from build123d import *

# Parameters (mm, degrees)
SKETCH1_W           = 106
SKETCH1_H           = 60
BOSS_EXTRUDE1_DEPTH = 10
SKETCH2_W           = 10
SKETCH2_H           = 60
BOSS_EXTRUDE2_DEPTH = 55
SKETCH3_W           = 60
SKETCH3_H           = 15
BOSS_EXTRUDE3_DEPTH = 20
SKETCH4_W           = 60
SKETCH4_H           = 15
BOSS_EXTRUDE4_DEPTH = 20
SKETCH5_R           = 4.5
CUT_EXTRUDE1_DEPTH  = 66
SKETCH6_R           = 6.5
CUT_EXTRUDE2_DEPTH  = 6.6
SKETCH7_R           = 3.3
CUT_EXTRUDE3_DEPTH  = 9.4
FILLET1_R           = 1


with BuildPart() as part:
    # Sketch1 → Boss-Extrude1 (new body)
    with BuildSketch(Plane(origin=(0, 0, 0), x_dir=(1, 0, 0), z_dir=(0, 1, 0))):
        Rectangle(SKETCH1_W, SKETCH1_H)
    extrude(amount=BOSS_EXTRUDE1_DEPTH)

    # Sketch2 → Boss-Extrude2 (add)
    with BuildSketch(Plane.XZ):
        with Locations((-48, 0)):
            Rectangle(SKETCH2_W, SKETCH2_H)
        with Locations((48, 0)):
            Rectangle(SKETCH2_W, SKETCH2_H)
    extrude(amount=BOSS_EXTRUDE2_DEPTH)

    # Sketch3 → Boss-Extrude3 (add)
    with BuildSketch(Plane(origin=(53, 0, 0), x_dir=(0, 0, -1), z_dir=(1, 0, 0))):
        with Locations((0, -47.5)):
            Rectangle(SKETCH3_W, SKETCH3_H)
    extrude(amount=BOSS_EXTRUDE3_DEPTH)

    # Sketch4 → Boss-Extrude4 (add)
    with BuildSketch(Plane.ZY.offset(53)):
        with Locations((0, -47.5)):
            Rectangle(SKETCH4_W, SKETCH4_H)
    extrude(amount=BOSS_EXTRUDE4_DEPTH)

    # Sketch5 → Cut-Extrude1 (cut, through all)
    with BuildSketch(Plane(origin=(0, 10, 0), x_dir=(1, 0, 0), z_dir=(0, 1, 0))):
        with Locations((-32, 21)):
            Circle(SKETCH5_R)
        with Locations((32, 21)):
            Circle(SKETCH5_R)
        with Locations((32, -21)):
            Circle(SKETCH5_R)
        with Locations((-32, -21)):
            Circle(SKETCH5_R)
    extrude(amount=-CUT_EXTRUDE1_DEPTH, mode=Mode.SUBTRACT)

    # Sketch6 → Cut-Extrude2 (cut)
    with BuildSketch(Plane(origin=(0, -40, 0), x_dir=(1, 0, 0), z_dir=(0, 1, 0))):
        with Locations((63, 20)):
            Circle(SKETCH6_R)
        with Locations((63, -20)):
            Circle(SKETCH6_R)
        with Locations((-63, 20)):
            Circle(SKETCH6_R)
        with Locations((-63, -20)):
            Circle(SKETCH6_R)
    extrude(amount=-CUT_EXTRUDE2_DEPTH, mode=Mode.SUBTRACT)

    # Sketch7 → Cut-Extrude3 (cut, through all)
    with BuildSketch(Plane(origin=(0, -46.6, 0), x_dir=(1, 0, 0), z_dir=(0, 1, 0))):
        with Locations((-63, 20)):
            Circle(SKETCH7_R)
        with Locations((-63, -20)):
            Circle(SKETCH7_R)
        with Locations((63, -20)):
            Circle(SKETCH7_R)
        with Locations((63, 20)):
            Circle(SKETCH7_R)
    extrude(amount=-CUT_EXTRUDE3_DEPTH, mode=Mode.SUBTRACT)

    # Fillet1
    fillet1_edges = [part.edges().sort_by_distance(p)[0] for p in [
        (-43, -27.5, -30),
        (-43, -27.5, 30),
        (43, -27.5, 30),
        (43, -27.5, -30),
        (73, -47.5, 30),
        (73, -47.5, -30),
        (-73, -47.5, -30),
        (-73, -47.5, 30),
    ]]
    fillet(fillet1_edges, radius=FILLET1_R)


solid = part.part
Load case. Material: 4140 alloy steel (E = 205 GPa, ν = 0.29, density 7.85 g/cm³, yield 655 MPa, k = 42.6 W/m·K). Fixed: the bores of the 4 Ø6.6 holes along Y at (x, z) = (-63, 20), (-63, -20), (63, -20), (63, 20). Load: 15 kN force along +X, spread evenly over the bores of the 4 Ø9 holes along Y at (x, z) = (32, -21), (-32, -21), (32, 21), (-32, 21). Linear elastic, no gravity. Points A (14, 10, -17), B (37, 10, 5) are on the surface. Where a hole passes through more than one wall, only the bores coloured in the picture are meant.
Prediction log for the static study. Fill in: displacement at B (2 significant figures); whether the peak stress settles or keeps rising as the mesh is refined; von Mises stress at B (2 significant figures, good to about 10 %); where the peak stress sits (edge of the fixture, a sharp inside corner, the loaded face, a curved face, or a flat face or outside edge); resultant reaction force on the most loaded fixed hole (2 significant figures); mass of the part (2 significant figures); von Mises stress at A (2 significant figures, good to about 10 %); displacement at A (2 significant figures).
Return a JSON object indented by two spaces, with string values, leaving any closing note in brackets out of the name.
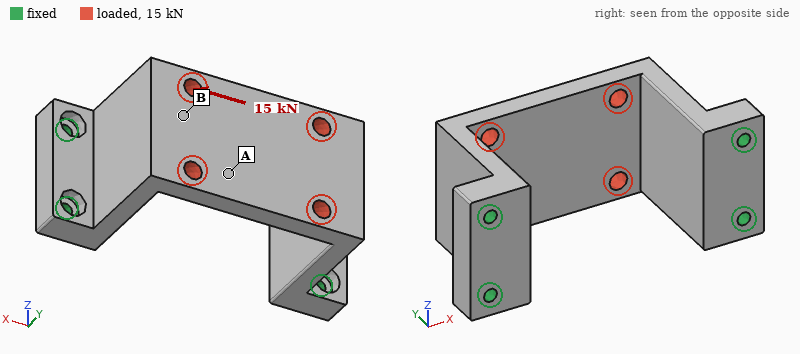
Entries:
{
  "displacement at B": "0.19 mm",
  "whether the peak stress settles or keeps rising as the mesh is refined": "keeps rising",
  "von Mises stress at B": "140 MPa",
  "where the peak stress sits": "edge of the fixture",
  "resultant reaction force on the most loaded fixed hole": "4.4 kN",
  "mass of the part": "1.2 kg",
  "von Mises stress at A": "52 MPa",
  "displacement at A": "0.18 mm"
}
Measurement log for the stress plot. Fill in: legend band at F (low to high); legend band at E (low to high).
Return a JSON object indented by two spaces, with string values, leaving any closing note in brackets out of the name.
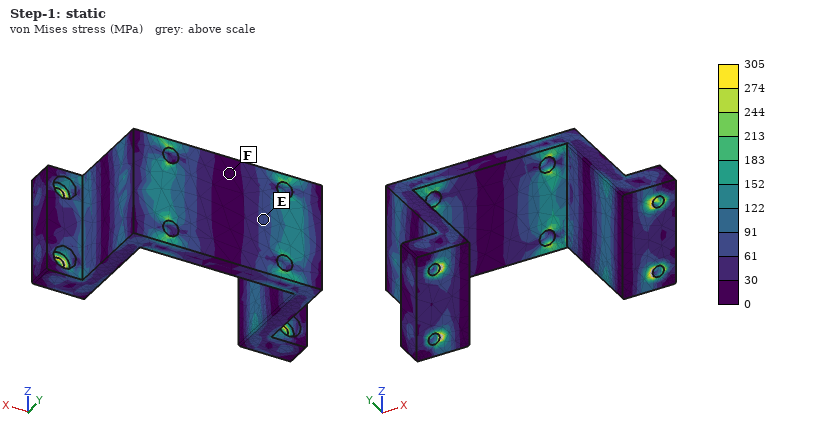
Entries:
{
  "legend band at F": "0 to 30 MPa",
  "legend band at E": "61 to 91 MPa"
}
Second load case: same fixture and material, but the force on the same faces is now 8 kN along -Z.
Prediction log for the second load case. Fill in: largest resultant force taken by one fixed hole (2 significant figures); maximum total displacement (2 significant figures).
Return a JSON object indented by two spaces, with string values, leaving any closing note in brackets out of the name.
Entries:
{
  "largest resultant force taken by one fixed hole": "5.8 kN",
  "maximum total displacement": "34 µm"
}
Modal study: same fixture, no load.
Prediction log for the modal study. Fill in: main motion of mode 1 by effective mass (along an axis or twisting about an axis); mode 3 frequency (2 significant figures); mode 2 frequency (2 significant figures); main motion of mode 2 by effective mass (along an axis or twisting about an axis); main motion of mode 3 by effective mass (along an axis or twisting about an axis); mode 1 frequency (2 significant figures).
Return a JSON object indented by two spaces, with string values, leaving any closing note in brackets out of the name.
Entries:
{
  "main motion of mode 1 by effective mass": "along X",
  "mode 3 frequency": "4100 Hz",
  "mode 2 frequency": "3300 Hz",
  "main motion of mode 2 by effective mass": "along Z",
  "main motion of mode 3 by effective mass": "twisting about Y",
  "mode 1 frequency": "1800 Hz"
}
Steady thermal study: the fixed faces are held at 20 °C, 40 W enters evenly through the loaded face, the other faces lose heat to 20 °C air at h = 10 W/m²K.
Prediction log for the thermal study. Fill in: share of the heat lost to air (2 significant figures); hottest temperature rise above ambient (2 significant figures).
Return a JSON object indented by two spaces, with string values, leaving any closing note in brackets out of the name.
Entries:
{
  "share of the heat lost to air": "24 %",
  "hottest temperature rise above ambient": "52 K"
}
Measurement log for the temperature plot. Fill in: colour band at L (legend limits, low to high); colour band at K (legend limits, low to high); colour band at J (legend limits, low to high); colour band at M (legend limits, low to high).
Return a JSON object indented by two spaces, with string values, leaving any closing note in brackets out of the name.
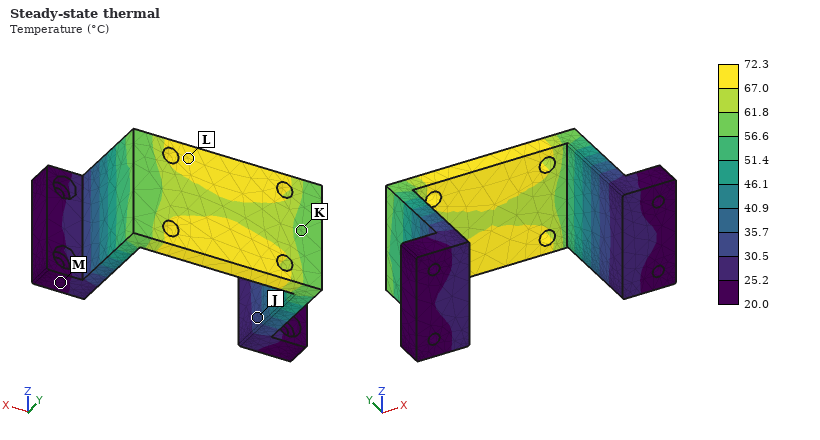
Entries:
{
  "colour band at L": "67.0 to 72.3 °C",
  "colour band at K": "56.6 to 61.8 °C",
  "colour band at J": "30.5 to 35.7 °C",
  "colour band at M": "20.0 to 25.2 °C"
}
